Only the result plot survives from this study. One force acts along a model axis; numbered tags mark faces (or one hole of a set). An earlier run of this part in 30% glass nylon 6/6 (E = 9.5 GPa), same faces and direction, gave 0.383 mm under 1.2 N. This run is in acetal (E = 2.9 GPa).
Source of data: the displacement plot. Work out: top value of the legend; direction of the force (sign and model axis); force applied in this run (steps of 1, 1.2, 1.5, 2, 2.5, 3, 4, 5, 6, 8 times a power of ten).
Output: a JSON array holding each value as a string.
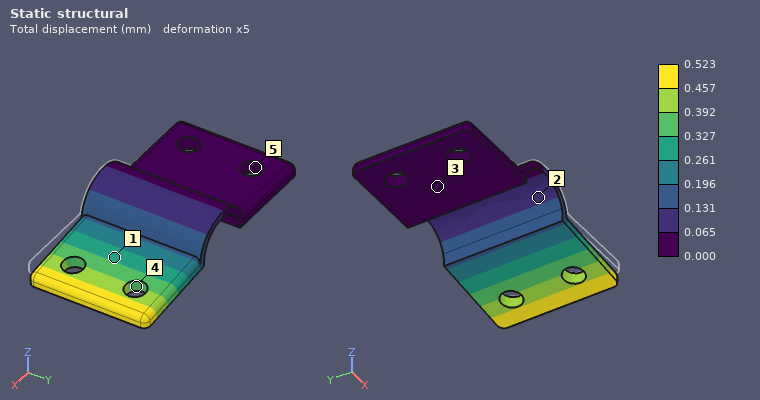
["0.523 mm", "-Z", "0.5 N"]
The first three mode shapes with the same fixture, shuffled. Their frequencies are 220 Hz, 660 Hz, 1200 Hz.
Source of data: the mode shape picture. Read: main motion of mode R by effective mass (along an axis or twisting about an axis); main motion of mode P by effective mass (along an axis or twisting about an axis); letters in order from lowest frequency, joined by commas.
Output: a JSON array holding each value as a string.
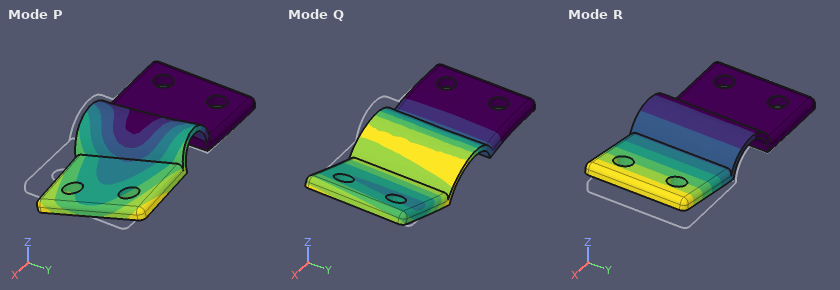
["along Z", "along Y", "R, P, Q"]
